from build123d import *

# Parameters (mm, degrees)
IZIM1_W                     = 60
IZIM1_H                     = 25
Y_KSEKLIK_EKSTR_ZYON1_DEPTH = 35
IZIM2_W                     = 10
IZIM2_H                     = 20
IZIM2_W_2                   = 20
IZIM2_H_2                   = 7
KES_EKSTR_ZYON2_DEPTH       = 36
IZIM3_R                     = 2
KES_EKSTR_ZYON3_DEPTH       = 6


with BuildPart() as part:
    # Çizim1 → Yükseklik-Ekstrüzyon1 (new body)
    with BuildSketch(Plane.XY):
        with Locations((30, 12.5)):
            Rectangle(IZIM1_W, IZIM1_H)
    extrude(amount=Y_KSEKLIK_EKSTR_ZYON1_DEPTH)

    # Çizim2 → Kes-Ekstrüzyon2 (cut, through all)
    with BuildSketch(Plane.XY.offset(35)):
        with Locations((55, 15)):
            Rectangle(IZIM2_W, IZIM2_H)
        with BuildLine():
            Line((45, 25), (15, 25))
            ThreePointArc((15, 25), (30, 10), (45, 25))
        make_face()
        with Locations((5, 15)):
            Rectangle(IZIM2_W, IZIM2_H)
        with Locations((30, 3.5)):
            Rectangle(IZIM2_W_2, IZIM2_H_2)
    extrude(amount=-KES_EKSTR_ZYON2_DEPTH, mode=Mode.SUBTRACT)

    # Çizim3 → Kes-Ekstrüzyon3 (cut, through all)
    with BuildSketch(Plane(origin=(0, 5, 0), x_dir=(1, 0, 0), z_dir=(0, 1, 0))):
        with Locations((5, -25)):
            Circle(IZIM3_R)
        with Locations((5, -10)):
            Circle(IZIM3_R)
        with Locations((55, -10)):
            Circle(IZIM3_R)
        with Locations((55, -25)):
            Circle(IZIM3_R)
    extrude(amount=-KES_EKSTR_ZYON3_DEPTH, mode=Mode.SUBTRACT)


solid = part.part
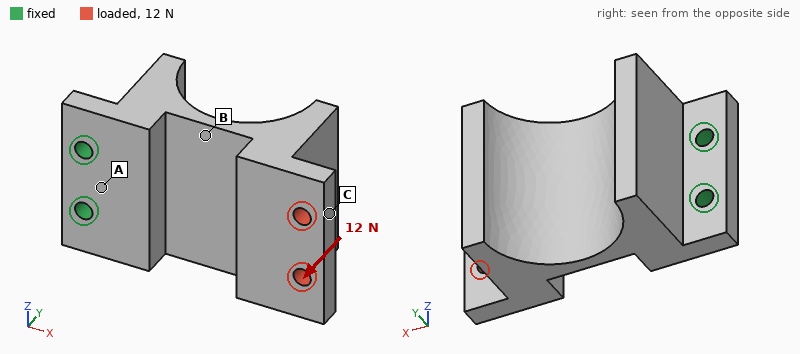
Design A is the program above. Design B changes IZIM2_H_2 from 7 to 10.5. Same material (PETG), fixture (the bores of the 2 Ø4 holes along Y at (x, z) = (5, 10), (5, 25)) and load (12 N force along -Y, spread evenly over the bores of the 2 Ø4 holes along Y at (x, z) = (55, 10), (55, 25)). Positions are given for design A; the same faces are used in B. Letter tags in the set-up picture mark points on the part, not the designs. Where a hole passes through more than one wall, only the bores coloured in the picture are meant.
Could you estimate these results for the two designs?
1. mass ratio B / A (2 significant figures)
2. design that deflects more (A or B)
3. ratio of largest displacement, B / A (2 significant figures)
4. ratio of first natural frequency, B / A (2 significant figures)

0.94
B
6.1
0.44
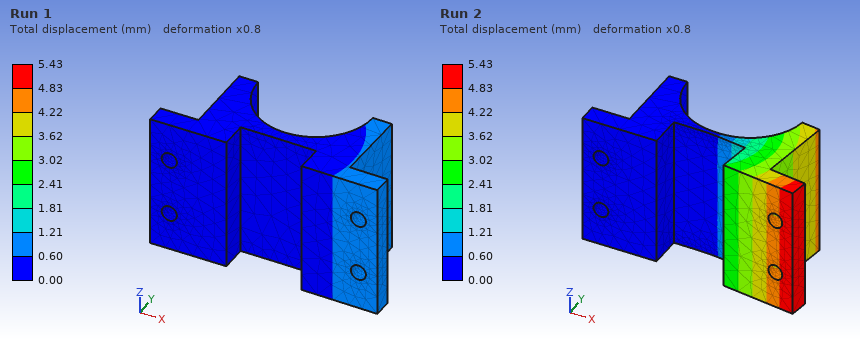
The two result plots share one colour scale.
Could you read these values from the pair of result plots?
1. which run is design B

Run 2
